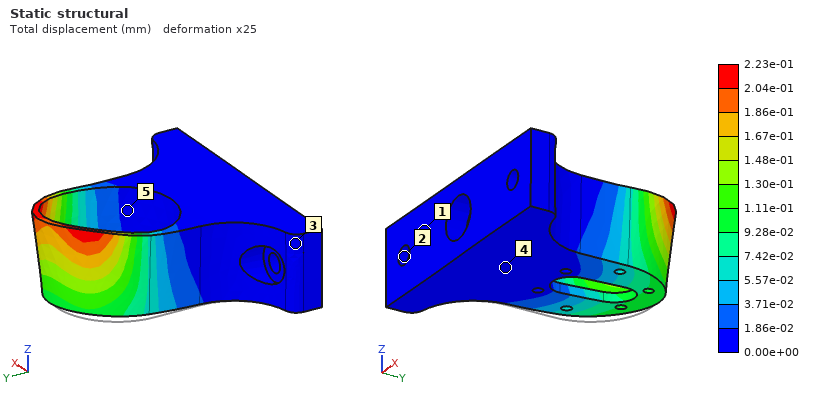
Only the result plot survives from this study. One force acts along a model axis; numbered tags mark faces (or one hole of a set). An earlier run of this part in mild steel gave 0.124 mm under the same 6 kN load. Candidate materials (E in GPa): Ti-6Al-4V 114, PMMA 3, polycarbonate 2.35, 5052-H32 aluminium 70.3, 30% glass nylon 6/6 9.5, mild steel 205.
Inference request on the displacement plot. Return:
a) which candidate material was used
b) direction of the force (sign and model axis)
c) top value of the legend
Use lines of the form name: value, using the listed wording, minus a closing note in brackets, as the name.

which candidate material was used: Ti-6Al-4V
direction of the force: +X
top value of the legend: 2.23e-01 mm
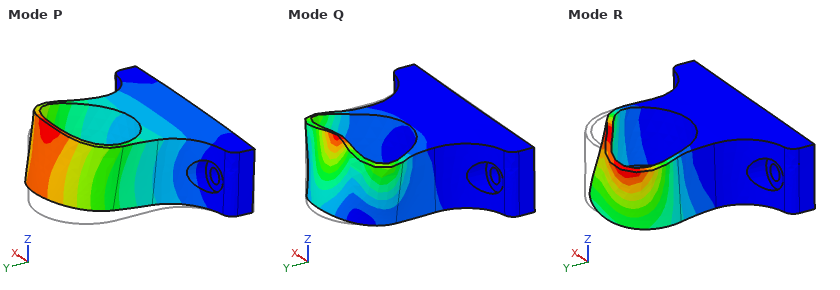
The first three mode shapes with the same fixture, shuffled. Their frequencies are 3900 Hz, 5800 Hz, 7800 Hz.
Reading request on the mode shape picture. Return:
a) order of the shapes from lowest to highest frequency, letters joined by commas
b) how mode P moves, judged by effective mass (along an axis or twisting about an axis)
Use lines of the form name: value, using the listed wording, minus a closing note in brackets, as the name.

order of the shapes from lowest to highest frequency, letters joined by commas: P, R, Q
how mode P moves, judged by effective mass: along Z
